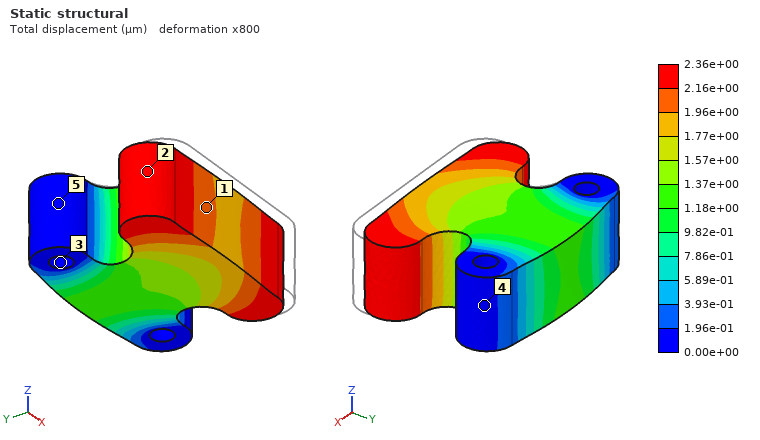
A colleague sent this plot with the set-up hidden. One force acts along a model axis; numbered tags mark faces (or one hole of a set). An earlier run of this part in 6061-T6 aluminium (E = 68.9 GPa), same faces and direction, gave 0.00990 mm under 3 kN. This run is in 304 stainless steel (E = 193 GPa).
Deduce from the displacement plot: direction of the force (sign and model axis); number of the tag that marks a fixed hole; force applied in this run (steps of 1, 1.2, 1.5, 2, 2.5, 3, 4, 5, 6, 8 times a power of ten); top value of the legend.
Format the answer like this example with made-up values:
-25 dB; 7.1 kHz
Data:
+Y; 3; 2 kN; 2.36e+00 µm
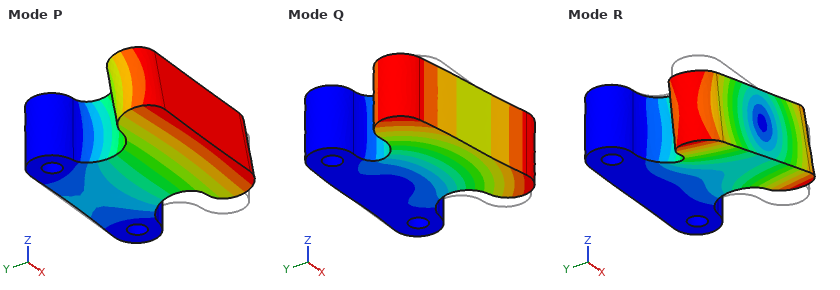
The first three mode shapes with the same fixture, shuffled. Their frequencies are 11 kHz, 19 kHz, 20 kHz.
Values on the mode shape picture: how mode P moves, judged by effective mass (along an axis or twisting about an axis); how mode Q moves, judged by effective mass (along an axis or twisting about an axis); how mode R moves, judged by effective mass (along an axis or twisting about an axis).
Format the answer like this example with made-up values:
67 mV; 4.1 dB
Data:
along Z; along X; twisting about Y
